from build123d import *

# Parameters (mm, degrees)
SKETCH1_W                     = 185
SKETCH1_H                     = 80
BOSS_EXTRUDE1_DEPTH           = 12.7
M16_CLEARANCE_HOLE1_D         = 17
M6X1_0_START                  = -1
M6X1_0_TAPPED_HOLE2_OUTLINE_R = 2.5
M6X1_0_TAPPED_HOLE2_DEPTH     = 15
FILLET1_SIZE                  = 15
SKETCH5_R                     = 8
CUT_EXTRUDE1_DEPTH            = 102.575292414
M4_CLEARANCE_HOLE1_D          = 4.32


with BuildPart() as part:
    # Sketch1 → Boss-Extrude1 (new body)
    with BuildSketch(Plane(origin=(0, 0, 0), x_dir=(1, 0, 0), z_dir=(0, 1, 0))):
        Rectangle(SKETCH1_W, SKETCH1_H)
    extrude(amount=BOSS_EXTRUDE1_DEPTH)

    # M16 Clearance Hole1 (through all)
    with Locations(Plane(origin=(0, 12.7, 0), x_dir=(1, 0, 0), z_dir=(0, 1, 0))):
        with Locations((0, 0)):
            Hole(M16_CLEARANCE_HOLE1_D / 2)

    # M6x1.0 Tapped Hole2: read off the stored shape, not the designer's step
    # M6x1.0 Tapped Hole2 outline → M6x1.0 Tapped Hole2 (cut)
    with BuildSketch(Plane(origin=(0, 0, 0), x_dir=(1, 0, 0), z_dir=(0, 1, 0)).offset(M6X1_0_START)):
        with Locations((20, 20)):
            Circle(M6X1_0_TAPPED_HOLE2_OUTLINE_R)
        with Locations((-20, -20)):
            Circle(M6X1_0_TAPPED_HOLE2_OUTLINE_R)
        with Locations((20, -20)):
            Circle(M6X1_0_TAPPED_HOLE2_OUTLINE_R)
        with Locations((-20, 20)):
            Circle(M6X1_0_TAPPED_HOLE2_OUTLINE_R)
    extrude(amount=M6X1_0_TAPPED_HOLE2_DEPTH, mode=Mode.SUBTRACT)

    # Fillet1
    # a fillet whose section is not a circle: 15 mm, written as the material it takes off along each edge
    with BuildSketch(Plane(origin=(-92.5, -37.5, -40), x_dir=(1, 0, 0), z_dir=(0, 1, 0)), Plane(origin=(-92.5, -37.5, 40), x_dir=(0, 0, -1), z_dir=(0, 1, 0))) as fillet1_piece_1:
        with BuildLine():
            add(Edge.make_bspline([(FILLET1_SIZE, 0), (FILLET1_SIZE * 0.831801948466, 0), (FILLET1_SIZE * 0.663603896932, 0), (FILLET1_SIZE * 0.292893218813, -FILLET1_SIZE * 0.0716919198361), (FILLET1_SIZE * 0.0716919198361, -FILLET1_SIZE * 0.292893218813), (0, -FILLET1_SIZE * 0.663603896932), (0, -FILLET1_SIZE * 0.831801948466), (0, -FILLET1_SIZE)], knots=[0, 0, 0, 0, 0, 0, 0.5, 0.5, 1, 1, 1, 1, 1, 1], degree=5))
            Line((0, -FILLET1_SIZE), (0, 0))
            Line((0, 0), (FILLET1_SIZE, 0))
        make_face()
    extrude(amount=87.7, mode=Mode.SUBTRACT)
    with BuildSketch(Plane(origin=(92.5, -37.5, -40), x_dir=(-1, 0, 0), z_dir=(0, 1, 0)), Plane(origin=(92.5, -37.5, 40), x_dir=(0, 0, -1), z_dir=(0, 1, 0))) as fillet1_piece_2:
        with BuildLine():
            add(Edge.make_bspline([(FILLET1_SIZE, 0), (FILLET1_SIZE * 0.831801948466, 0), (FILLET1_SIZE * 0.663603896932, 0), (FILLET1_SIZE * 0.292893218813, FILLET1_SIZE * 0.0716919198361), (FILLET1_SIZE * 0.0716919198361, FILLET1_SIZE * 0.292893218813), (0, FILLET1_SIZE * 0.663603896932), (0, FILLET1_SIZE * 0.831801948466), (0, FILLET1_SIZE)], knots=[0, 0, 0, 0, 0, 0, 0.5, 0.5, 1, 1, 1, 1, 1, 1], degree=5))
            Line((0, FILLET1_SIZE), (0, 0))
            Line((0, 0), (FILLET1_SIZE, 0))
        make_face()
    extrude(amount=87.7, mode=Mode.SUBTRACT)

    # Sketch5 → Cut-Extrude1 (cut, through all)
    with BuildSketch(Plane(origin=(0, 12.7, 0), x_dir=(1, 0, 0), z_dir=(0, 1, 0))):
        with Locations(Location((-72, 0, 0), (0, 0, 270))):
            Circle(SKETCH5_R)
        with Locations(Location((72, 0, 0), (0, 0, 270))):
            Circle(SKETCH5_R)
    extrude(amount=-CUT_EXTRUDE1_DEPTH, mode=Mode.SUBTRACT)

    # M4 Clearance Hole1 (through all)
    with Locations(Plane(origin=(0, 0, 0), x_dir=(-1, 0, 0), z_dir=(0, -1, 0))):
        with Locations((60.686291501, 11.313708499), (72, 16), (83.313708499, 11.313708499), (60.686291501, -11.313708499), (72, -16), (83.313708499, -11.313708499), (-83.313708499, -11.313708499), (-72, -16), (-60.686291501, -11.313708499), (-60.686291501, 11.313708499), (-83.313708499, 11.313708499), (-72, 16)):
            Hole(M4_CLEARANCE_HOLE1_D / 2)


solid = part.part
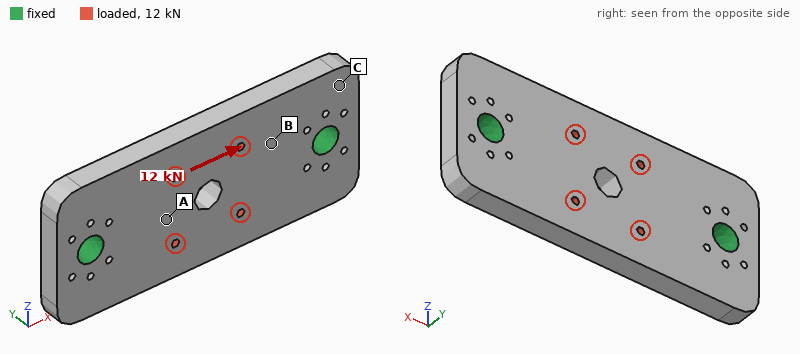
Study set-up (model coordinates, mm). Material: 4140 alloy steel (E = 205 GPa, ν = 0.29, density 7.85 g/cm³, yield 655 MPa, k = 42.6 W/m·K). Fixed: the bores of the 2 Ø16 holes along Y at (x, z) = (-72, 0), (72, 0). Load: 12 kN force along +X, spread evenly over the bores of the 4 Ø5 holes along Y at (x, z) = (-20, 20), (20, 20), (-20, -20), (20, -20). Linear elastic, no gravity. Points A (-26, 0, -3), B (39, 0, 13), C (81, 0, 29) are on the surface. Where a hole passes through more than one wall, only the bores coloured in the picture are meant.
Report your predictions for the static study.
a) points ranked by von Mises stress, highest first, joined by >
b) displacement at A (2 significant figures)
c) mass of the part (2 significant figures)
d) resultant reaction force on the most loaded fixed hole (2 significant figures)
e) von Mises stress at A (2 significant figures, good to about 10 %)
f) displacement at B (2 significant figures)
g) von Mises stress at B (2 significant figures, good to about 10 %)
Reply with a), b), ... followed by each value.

a) B > A > C
b) 1.9 µm
c) 1.4 kg
d) 6.0 kN
e) 4.8 MPa
f) 1.7 µm
g) 8.9 MPa
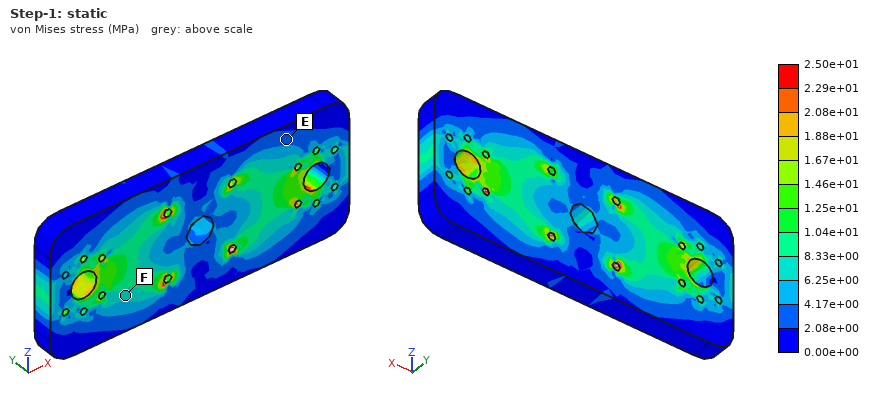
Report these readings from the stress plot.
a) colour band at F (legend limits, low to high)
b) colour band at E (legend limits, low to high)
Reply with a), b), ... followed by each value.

a) 6.25e+00 to 8.33e+00 MPa
b) 2.08e+00 to 4.17e+00 MPa
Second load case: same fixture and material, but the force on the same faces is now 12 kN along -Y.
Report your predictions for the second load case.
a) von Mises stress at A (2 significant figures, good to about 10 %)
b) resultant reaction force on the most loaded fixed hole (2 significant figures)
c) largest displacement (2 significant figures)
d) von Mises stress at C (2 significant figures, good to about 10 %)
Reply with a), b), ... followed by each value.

a) 37 MPa
b) 6.0 kN
c) 71 µm
d) 21 MPa
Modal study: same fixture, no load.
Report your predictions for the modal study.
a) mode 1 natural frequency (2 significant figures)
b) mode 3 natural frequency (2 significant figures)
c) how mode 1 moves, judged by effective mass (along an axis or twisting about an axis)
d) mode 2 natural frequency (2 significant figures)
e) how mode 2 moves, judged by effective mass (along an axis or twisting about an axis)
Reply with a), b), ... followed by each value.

a) 2900 Hz
b) 6400 Hz
c) along Y
d) 3300 Hz
e) twisting about X
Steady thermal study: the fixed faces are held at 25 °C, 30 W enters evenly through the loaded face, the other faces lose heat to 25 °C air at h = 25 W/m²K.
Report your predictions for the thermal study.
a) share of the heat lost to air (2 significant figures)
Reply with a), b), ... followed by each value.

a) 26 %
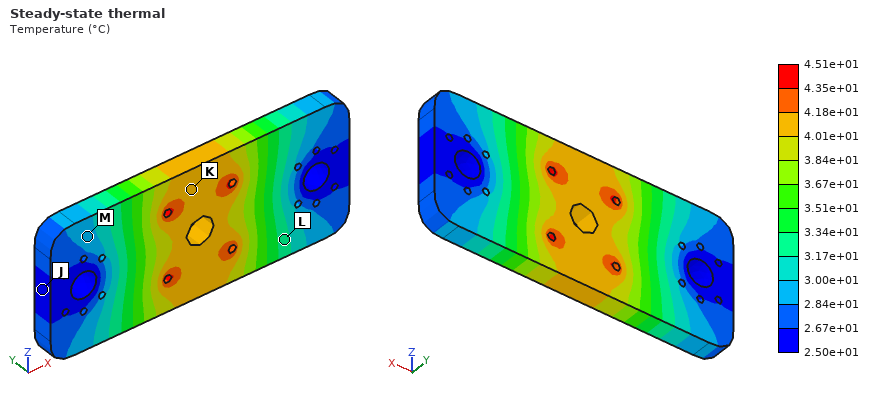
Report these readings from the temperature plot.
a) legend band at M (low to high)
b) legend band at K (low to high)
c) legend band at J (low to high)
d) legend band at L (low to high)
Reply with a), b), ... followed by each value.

a) 2.84e+01 to 3.00e+01 °C
b) 4.01e+01 to 4.18e+01 °C
c) 2.50e+01 to 2.67e+01 °C
d) 3.17e+01 to 3.34e+01 °C
